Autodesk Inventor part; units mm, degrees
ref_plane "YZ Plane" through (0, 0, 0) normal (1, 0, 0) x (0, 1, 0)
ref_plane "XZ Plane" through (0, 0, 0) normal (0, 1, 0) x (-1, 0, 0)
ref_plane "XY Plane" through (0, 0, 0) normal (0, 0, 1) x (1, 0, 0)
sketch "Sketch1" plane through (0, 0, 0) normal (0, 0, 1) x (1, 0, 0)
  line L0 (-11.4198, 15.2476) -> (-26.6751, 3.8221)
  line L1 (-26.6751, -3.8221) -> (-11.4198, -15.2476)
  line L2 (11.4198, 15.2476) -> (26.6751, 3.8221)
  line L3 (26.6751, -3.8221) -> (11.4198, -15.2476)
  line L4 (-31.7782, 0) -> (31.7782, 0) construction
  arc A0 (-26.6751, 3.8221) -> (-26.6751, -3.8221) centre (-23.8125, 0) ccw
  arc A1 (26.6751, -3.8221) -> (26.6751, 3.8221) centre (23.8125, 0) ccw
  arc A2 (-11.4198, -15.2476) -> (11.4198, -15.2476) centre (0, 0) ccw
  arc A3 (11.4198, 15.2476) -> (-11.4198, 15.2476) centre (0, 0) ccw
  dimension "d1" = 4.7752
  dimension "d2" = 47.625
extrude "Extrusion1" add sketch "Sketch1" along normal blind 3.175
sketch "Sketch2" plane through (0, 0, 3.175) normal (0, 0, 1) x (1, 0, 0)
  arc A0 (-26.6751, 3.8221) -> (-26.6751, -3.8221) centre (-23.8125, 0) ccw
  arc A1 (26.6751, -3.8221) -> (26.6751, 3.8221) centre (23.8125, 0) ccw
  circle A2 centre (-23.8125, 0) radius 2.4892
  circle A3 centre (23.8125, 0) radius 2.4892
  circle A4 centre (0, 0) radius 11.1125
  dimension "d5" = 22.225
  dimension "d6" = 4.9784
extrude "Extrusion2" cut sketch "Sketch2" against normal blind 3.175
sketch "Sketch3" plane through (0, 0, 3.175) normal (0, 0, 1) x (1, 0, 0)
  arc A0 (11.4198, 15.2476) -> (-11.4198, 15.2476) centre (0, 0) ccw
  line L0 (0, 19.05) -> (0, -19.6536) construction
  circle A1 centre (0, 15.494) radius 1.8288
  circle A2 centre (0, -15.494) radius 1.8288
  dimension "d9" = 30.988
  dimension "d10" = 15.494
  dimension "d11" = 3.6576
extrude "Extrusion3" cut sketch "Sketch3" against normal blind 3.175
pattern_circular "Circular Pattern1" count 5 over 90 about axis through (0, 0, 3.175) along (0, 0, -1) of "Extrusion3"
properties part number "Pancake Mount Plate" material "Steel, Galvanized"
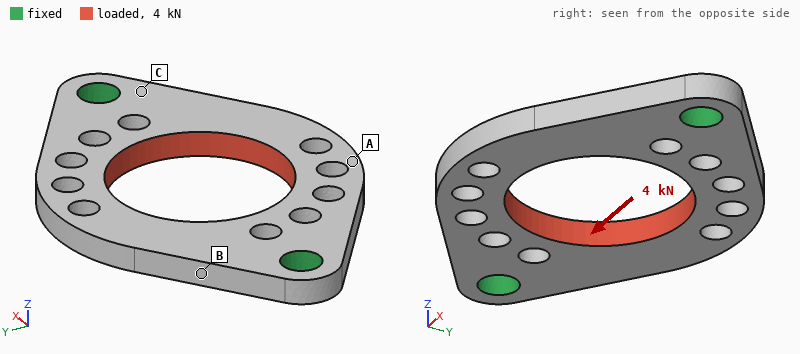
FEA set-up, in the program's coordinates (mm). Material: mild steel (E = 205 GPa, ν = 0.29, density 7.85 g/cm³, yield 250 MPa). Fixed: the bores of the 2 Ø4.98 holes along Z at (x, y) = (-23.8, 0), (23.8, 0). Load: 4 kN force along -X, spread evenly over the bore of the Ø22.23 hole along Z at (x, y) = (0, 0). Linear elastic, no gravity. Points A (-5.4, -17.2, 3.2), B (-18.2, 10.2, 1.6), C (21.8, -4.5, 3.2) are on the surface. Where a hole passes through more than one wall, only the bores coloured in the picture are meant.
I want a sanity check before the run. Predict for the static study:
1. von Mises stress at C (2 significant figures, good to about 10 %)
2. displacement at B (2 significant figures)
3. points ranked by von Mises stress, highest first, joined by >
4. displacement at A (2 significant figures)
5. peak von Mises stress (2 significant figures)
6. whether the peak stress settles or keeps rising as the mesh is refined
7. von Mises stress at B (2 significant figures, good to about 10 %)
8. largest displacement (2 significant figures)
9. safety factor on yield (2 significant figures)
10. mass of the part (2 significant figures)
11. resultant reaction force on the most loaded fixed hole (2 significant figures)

51 MPa
4.3 µm
C > B > A
5.1 µm
170 MPa
settles
27 MPa
7.3 µm
1.4
22 g
2.0 kN
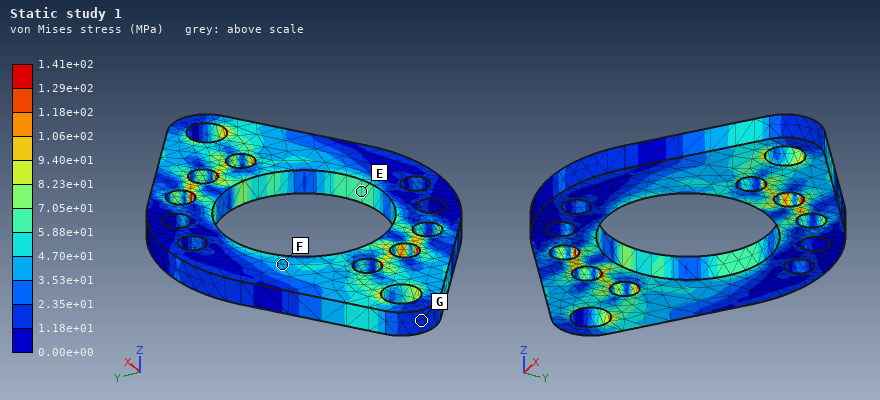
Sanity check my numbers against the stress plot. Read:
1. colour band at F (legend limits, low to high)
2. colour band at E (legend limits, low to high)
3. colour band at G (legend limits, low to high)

3.53e+01 to 4.70e+01 MPa
5.88e+01 to 7.05e+01 MPa
1.18e+01 to 2.35e+01 MPa
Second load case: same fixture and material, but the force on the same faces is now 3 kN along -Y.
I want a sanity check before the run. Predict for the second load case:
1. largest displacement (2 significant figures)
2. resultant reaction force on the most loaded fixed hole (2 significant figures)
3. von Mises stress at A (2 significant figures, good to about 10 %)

9.6 µm
1.5 kN
62 MPa
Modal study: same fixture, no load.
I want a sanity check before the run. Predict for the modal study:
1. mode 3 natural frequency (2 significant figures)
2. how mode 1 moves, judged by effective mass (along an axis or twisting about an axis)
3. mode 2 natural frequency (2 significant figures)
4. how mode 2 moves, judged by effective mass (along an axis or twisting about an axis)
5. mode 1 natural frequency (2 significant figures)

14 kHz
twisting about X
5500 Hz
along Z
5000 Hz
